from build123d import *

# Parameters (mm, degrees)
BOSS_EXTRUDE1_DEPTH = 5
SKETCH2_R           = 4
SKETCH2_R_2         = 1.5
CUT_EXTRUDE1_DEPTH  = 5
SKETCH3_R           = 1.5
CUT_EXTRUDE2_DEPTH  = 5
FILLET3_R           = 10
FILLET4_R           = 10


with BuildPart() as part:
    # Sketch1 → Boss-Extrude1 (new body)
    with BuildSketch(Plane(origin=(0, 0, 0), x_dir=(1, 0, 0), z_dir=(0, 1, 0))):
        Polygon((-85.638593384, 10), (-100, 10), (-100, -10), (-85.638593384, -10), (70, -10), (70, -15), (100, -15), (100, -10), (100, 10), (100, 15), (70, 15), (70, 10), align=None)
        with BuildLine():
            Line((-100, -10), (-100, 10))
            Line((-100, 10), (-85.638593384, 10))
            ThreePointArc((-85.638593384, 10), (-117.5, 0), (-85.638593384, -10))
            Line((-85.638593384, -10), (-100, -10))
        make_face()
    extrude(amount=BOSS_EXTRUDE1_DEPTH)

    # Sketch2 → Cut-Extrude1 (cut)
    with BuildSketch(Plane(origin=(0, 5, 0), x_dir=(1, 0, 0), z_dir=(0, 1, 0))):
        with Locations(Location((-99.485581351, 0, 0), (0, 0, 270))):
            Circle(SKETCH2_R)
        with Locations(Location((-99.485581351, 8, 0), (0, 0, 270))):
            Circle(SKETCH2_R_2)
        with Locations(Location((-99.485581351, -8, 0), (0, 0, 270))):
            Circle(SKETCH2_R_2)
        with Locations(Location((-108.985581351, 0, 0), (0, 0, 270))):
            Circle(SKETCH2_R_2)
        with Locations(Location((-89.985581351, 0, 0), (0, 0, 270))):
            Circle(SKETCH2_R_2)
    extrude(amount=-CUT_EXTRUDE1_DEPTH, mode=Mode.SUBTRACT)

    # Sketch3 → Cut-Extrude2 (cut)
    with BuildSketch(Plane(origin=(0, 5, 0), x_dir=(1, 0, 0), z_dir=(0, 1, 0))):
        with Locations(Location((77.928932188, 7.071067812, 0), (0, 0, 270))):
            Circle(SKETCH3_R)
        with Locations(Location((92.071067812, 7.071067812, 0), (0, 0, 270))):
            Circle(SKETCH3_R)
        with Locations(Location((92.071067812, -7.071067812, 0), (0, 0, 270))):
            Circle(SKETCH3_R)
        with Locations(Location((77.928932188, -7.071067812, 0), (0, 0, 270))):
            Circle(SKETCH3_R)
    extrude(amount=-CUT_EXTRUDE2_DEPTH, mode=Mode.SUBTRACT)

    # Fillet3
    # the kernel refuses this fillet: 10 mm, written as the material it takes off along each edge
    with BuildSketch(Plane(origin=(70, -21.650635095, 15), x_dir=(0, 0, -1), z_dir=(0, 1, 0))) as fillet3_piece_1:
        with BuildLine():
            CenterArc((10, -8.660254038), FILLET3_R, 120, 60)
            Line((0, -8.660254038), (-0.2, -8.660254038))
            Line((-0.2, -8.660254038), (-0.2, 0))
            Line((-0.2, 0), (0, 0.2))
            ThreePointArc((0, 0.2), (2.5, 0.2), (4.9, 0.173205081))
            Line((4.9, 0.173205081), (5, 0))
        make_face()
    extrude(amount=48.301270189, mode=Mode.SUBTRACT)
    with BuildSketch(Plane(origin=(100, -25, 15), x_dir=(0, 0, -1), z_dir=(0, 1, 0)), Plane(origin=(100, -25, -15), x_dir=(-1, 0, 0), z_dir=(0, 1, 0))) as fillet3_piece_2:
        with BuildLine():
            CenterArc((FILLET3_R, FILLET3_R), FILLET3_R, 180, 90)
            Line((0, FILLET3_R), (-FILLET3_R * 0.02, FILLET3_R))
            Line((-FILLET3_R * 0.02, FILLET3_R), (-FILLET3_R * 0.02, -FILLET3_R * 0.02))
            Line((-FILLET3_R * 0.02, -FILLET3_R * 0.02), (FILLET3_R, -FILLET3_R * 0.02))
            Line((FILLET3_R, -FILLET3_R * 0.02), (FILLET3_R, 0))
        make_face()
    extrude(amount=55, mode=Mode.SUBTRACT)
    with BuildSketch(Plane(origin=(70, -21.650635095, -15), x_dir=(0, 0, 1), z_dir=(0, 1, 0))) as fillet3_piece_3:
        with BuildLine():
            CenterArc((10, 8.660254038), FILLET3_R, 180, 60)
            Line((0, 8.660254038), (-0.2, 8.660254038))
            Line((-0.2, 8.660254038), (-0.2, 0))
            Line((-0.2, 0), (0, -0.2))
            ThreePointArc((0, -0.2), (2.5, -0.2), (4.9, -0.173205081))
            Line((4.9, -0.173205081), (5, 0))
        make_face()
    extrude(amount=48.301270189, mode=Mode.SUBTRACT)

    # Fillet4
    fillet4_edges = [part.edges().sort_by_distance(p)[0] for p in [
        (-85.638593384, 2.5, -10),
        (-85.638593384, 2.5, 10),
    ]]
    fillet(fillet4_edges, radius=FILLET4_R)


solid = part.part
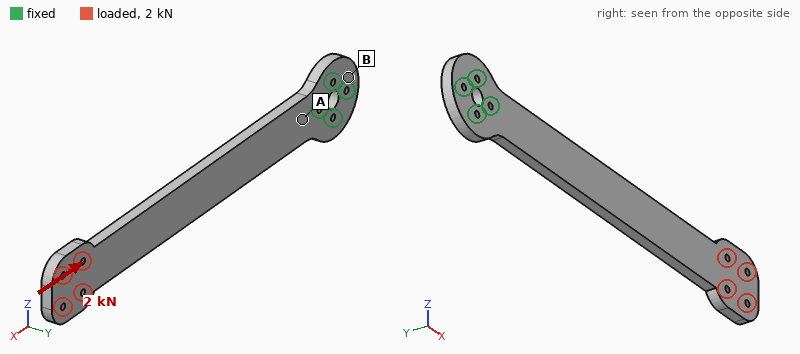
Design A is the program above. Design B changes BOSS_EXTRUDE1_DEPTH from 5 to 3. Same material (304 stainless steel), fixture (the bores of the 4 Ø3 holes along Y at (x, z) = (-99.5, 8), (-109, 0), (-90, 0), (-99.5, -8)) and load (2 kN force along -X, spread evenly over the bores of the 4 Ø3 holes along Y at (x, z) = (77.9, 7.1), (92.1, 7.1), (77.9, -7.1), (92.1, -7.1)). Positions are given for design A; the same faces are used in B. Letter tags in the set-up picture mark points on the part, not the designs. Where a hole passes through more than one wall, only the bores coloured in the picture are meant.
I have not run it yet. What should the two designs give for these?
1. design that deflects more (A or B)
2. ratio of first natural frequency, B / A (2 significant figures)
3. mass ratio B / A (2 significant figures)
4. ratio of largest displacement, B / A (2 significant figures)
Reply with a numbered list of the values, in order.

1. B
2. 0.60
3. 0.60
4. 1.7
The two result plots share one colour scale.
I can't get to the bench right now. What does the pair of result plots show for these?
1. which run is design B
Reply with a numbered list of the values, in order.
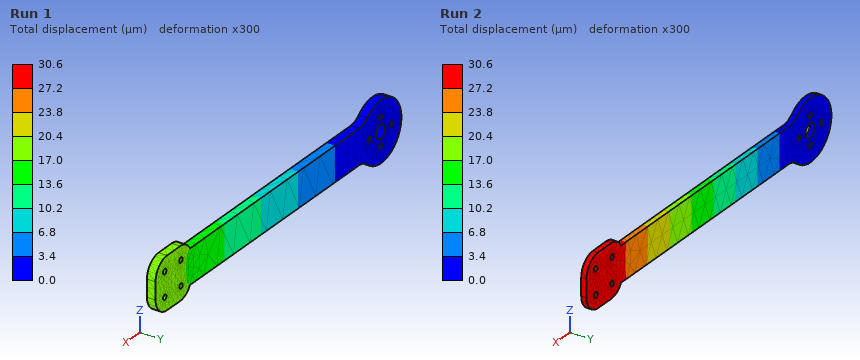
1. Run 2
